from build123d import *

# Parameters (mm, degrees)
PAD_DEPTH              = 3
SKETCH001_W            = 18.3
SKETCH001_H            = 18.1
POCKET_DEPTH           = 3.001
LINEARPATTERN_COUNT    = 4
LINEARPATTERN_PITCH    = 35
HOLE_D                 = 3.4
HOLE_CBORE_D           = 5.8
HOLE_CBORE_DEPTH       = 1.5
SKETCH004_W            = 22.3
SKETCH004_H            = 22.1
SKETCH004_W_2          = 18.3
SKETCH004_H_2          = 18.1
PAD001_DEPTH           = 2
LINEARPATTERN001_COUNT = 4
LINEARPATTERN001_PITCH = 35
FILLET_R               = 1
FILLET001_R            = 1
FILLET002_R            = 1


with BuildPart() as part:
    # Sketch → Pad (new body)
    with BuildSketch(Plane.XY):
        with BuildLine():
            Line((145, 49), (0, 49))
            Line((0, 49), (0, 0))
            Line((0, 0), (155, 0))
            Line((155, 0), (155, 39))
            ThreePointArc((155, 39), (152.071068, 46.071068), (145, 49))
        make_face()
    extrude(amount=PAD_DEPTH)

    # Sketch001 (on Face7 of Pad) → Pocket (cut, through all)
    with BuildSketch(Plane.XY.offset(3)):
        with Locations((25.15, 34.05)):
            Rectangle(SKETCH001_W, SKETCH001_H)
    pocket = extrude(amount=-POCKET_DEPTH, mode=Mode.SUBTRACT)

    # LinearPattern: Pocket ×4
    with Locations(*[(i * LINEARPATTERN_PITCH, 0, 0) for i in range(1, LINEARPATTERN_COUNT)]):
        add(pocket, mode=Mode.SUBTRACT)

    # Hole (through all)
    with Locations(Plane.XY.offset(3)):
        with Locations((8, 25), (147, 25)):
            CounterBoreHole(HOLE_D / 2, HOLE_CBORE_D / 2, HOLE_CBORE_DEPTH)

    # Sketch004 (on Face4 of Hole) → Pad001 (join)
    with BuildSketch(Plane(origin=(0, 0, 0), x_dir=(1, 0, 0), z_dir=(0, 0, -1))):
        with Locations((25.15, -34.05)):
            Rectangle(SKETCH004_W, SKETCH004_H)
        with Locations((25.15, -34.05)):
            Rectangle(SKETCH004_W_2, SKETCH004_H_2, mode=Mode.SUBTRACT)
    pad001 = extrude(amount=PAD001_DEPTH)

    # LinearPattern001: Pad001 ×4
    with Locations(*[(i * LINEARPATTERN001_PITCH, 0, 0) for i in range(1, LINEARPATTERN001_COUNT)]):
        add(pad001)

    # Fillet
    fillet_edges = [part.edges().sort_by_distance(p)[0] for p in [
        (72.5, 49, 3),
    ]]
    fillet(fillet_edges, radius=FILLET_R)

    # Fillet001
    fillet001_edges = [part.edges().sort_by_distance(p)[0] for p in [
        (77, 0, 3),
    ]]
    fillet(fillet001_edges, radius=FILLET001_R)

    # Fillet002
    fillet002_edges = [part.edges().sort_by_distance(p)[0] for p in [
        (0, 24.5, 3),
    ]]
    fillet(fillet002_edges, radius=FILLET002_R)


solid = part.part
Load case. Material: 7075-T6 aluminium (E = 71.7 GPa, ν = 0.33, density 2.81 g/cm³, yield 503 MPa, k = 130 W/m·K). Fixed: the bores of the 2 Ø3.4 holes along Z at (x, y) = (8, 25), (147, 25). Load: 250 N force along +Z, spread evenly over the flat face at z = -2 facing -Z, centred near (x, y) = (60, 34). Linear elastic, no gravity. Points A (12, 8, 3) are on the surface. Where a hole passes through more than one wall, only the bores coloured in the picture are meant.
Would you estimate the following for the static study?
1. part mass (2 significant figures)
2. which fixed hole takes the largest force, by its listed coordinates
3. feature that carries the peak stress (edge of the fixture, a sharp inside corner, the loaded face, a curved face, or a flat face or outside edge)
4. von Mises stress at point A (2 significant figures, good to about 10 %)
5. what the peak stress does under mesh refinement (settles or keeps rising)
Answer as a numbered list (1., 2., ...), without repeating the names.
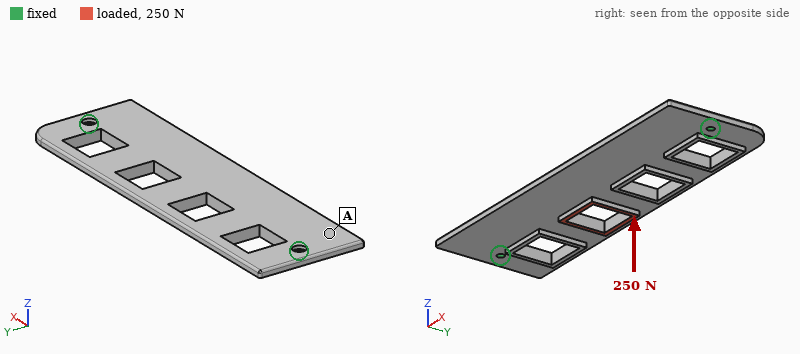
1. 56 g
2. (8, 25)
3. edge of the fixture
4. 23 MPa
5. keeps rising
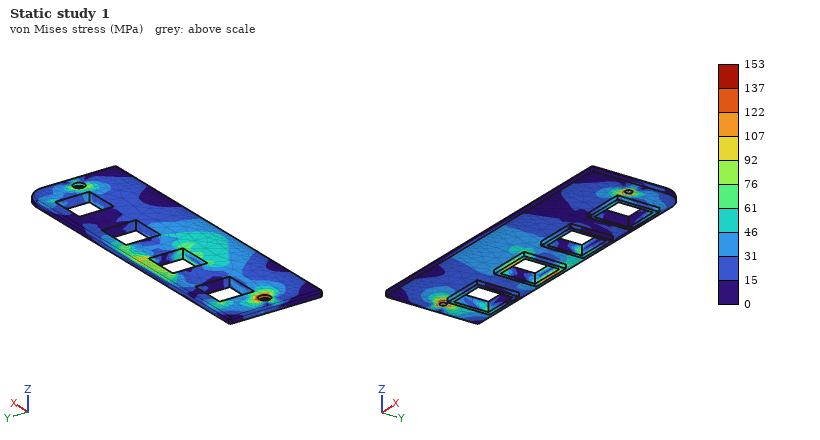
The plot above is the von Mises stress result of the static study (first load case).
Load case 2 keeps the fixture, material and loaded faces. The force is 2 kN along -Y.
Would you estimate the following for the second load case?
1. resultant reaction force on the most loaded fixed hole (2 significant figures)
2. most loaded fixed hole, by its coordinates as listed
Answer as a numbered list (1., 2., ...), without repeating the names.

1. 1.4 kN
2. (8, 25)
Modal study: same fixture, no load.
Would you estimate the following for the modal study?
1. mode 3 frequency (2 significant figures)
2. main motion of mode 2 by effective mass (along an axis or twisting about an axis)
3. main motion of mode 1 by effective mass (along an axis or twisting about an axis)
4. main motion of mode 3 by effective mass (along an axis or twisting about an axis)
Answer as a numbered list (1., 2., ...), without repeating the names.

1. 1700 Hz
2. twisting about X
3. along Z
4. twisting about Y
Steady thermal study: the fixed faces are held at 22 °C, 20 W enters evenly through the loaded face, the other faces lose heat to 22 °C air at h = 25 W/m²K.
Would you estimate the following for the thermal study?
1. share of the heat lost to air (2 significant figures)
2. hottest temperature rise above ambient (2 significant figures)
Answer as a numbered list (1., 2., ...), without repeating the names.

1. 39 %
2. 49 K
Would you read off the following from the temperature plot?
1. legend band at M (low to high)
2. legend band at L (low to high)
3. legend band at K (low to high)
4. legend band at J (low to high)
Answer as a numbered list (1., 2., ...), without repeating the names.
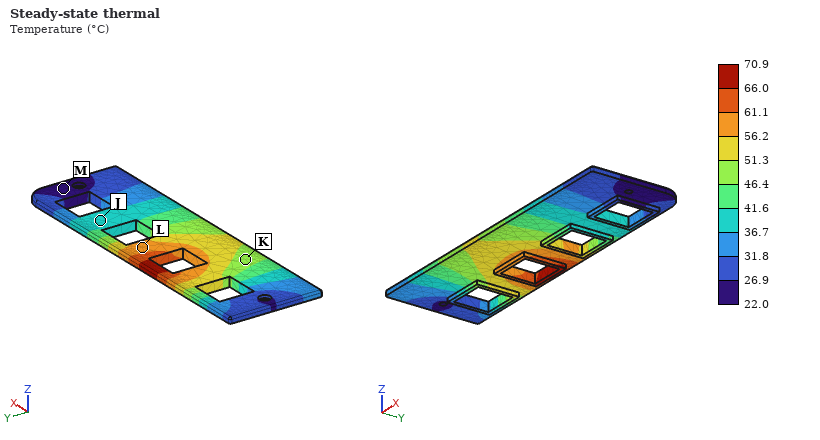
1. 22.0 to 26.9 °C
2. 56.2 to 61.1 °C
3. 46.4 to 51.3 °C
4. 36.7 to 41.6 °C
